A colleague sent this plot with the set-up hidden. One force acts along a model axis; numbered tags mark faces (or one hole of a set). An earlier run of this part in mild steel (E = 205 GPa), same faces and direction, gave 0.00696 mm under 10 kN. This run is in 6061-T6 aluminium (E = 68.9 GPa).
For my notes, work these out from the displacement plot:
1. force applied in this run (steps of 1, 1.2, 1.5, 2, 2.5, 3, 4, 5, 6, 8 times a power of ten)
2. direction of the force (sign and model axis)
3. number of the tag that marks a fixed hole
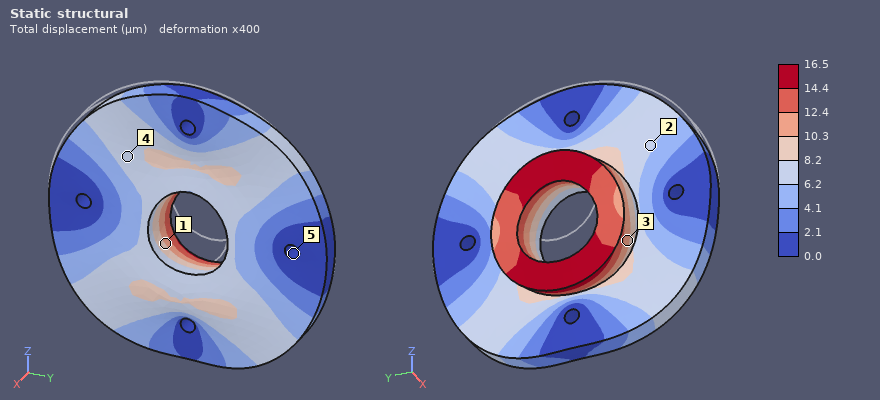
8 kN
-Z
5
